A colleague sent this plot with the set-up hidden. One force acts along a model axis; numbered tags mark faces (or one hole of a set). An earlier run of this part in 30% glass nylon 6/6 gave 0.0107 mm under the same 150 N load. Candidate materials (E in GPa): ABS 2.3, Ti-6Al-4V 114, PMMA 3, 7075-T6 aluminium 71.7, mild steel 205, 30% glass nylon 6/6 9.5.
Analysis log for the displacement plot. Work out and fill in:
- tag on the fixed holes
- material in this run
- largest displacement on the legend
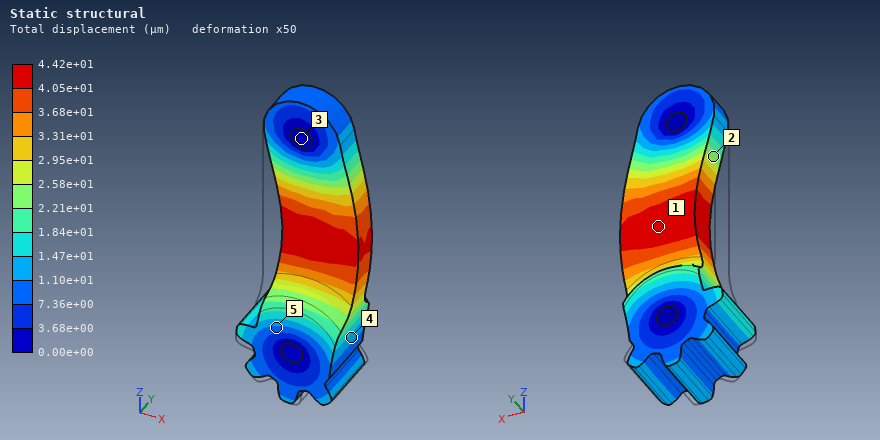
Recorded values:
3
ABS
4.42e+01 µm
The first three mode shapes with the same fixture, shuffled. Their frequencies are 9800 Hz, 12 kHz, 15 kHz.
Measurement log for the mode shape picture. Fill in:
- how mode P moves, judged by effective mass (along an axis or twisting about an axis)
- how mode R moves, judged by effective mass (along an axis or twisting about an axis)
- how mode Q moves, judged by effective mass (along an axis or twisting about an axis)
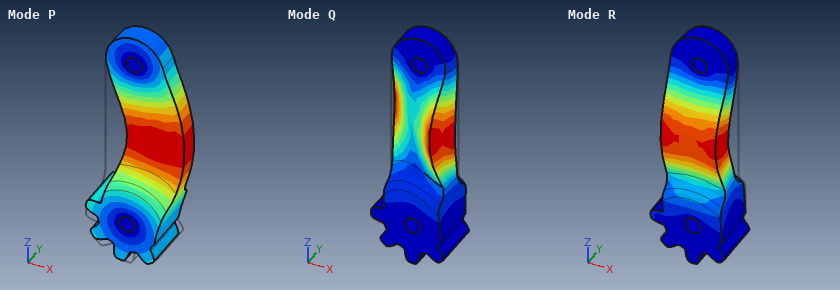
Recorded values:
along X
along Y
twisting about Z
